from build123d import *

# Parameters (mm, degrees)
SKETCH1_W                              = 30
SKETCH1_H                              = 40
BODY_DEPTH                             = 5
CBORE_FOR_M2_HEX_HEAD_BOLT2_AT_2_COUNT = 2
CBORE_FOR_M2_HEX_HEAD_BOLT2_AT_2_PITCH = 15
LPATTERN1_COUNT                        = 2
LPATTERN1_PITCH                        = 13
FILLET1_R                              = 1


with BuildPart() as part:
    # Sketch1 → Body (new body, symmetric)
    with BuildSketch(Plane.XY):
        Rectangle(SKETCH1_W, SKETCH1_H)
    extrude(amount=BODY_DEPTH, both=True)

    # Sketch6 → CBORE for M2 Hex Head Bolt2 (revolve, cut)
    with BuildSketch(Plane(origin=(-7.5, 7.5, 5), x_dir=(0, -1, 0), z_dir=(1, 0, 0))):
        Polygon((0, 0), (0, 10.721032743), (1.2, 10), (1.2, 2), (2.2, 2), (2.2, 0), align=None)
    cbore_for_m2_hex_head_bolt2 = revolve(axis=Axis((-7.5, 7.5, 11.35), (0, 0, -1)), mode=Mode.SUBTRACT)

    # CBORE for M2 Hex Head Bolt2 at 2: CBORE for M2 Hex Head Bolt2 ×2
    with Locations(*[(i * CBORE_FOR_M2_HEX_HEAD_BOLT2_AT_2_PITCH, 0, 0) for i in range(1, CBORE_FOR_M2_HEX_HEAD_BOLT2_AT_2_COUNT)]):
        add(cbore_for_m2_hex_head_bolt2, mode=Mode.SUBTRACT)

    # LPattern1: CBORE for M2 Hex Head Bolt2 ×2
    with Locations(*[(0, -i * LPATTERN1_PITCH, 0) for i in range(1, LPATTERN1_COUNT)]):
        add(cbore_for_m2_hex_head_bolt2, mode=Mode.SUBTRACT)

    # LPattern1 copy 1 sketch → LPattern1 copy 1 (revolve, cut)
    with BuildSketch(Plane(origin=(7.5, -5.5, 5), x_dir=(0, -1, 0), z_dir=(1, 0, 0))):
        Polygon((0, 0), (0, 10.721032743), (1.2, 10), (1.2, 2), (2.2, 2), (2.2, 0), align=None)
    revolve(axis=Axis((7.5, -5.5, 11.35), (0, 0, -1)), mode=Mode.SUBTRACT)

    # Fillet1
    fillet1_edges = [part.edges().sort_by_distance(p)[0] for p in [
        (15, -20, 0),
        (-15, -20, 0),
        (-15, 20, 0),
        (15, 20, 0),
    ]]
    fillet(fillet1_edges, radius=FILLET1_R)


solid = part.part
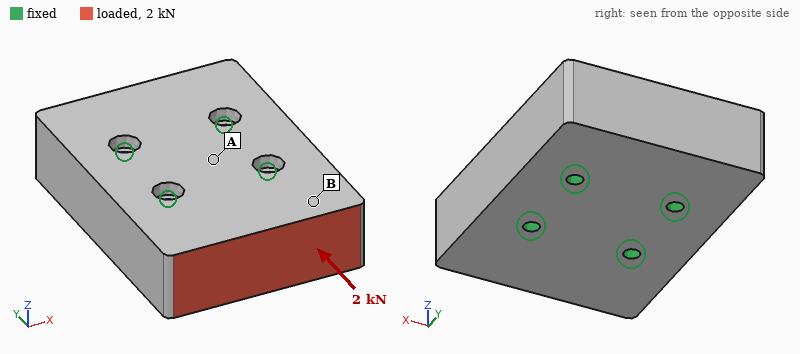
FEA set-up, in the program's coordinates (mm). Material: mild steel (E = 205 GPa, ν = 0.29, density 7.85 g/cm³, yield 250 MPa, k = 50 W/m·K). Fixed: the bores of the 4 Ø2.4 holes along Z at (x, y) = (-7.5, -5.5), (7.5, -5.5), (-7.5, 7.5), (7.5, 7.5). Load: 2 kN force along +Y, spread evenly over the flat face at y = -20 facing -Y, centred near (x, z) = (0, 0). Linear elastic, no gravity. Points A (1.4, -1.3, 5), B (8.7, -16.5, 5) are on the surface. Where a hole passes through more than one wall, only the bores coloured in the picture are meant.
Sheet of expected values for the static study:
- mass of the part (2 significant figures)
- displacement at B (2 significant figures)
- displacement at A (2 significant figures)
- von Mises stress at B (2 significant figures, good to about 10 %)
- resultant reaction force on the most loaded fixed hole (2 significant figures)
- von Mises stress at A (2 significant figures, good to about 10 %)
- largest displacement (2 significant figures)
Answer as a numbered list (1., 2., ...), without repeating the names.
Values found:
1. 92 g
2. 0.63 µm
3. 0.16 µm
4. 7.5 MPa
5. 780 N
6. 4.0 MPa
7. 0.76 µm
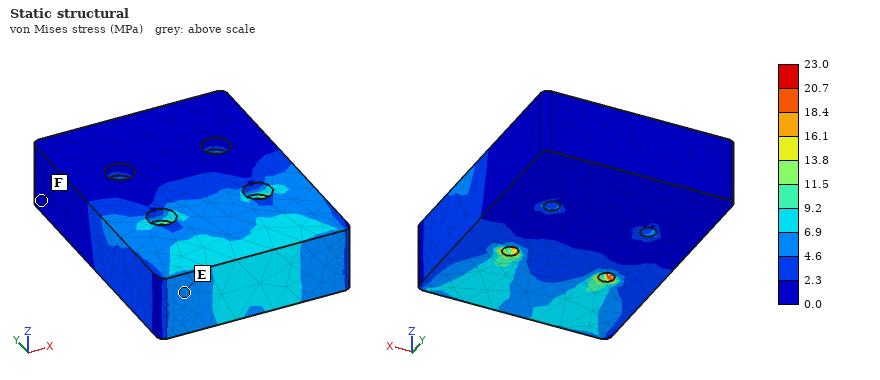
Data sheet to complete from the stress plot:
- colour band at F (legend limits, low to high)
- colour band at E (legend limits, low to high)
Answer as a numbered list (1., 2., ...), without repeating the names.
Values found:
1. 0.0 to 2.3 MPa
2. 4.6 to 6.9 MPa
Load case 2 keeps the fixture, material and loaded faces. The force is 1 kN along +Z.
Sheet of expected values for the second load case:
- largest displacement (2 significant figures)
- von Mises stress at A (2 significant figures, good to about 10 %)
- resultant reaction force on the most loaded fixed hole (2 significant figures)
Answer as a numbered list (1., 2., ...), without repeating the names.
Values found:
1. 4.6 µm
2. 13 MPa
3. 730 N
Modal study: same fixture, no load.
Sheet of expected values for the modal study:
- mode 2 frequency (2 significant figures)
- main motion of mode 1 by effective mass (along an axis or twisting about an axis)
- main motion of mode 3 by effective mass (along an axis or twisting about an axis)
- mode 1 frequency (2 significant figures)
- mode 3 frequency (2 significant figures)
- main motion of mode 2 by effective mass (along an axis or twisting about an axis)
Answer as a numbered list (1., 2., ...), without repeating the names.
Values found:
1. 29 kHz
2. along Z
3. twisting about Y
4. 23 kHz
5. 32 kHz
6. along Z
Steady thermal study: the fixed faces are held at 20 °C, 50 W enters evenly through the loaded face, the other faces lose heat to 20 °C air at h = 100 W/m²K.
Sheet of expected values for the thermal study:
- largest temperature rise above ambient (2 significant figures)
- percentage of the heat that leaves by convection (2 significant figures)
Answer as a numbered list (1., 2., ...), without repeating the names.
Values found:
1. 54 K
2. 7.9 %
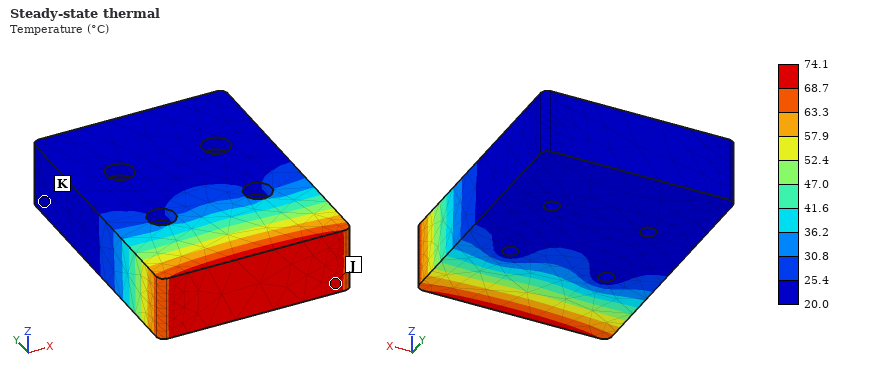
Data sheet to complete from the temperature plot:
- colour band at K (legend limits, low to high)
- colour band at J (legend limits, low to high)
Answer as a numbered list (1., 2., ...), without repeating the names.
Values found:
1. 20.0 to 25.4 °C
2. 68.7 to 74.1 °C
